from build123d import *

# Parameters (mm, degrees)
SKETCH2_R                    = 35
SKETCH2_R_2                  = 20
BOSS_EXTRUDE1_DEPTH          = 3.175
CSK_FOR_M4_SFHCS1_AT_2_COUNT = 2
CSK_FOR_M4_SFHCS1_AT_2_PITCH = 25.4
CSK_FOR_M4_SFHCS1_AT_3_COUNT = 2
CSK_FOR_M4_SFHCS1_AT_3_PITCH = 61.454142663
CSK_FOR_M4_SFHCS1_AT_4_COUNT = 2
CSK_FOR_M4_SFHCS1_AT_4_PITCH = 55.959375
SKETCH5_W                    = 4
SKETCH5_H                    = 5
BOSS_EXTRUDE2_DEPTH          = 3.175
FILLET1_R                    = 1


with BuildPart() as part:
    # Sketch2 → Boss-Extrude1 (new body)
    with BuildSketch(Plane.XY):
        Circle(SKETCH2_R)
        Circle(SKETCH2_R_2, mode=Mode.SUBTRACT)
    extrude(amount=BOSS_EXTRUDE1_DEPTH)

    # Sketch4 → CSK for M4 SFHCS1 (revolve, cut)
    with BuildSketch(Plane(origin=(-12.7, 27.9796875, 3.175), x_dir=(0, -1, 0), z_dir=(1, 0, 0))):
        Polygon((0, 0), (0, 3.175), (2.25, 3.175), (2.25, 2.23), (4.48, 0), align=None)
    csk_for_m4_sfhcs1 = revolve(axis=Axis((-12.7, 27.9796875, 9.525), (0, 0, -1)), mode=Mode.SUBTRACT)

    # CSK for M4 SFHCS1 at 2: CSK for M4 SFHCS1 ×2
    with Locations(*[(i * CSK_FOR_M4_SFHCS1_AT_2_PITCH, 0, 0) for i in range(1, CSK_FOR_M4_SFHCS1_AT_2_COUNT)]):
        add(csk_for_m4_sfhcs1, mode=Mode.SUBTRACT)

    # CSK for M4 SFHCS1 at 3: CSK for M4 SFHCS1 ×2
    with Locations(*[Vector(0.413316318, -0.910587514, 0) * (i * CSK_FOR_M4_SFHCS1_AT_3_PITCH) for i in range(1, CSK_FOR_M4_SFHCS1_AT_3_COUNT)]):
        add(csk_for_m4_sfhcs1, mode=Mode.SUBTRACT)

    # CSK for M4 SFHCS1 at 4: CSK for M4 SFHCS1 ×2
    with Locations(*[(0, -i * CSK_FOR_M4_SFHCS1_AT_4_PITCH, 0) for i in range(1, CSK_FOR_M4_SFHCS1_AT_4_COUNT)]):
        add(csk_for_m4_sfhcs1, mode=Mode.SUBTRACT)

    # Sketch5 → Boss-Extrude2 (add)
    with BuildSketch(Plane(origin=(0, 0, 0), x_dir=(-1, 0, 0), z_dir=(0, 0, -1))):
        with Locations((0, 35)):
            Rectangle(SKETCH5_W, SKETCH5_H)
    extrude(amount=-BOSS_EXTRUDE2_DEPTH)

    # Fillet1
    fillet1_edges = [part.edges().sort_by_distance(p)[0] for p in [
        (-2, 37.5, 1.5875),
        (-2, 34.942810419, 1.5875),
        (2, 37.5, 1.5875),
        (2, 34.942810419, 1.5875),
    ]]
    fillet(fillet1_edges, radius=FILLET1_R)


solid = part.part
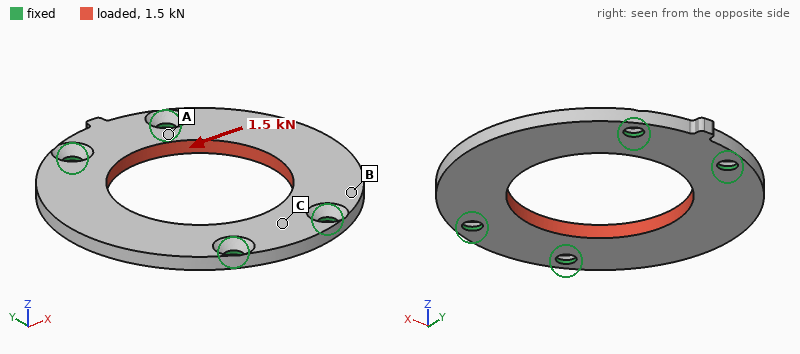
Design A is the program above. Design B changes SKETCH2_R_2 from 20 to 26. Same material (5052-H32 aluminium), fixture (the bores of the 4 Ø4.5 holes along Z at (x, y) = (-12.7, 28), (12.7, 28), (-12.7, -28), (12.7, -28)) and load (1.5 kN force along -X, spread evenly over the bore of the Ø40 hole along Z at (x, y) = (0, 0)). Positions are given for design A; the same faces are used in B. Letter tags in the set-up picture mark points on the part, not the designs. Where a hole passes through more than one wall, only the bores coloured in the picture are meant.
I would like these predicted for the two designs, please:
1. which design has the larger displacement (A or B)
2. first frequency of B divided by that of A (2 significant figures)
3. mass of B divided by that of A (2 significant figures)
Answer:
B
0.85
0.65
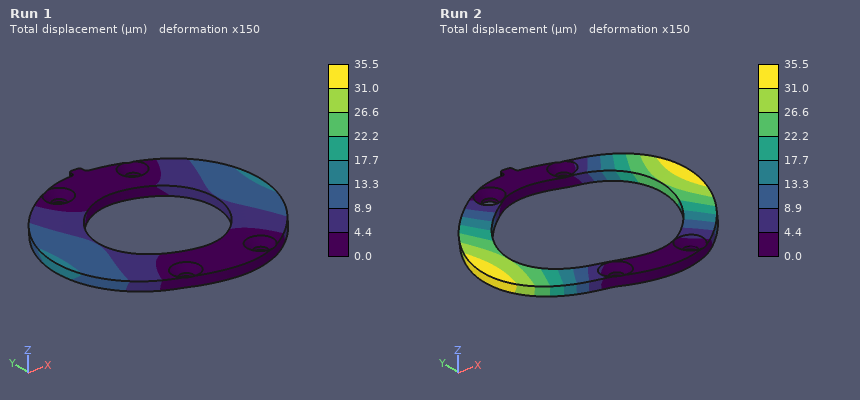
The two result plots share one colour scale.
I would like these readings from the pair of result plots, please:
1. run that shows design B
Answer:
Run 2
